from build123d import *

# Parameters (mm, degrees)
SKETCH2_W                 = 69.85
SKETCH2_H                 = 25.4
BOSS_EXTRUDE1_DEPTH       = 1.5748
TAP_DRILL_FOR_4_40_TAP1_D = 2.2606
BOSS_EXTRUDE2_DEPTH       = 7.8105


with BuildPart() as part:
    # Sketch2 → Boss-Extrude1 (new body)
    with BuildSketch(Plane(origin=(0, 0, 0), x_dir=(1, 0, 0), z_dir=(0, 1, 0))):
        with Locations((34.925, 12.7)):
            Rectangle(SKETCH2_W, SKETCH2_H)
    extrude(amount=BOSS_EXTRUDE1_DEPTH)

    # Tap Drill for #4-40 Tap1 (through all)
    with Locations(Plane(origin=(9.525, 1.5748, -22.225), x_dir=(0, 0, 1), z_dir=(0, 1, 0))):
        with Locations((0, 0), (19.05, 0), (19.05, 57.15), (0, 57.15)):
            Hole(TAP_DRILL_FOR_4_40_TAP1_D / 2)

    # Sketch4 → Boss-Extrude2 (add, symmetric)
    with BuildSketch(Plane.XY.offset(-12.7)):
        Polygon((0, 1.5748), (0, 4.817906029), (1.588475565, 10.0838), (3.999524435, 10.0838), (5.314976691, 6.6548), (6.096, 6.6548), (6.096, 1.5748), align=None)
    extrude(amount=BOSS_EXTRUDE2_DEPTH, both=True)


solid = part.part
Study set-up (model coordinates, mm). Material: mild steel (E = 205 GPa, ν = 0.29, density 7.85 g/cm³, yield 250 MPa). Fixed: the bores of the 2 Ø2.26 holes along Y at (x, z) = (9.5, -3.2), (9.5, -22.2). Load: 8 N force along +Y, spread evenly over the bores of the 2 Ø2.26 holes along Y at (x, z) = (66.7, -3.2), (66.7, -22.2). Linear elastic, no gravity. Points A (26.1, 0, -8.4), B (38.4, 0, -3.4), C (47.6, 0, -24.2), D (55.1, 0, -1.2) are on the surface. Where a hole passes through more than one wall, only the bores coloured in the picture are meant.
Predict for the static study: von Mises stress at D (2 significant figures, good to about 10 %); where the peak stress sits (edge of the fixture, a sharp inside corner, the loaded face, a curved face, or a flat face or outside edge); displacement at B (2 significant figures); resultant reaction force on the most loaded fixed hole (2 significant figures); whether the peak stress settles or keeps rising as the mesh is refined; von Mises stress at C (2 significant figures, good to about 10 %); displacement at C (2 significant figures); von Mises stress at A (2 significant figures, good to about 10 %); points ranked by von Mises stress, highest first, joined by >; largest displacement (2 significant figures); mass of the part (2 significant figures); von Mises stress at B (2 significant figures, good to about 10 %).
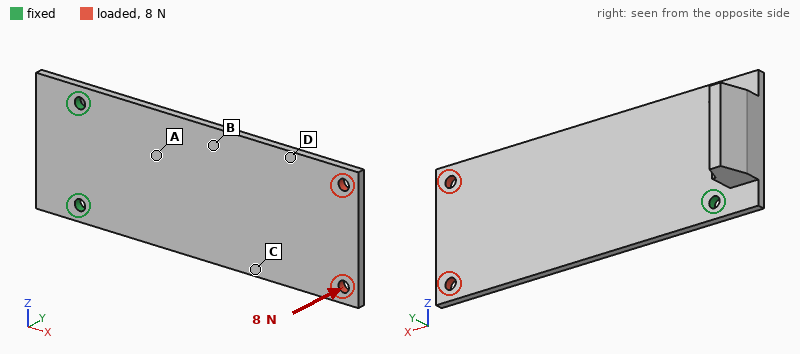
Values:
9.4 MPa
edge of the fixture
0.095 mm
4.4 N
keeps rising
15 MPa
0.15 mm
30 MPa
A > B > C > D
0.32 mm
27 g
22 MPa
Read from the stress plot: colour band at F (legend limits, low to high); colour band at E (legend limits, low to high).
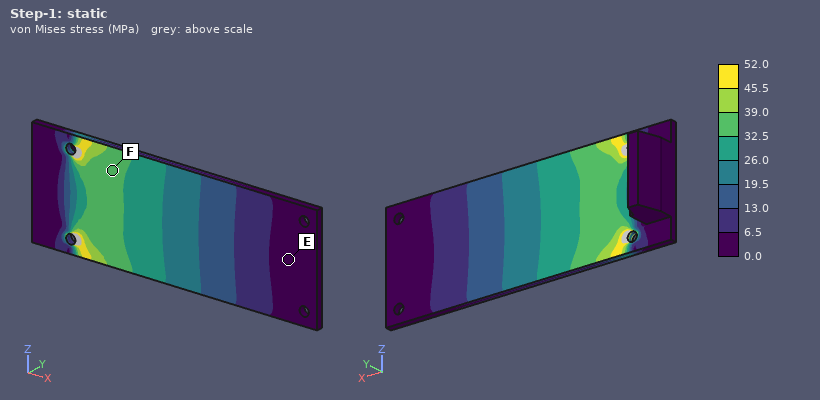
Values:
32.5 to 39.0 MPa
0.0 to 6.5 MPa
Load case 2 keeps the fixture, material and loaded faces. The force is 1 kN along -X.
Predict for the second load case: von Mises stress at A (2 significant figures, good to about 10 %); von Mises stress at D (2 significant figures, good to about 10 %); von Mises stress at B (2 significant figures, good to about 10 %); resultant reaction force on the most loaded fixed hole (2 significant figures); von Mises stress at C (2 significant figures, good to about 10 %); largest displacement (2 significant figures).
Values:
24 MPa
31 MPa
25 MPa
500 N
26 MPa
9.0 µm
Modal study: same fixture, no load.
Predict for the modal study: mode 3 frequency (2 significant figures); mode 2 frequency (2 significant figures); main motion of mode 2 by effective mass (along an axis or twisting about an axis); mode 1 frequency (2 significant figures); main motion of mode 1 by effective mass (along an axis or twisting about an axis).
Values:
2200 Hz
1800 Hz
twisting about X
360 Hz
along Y
